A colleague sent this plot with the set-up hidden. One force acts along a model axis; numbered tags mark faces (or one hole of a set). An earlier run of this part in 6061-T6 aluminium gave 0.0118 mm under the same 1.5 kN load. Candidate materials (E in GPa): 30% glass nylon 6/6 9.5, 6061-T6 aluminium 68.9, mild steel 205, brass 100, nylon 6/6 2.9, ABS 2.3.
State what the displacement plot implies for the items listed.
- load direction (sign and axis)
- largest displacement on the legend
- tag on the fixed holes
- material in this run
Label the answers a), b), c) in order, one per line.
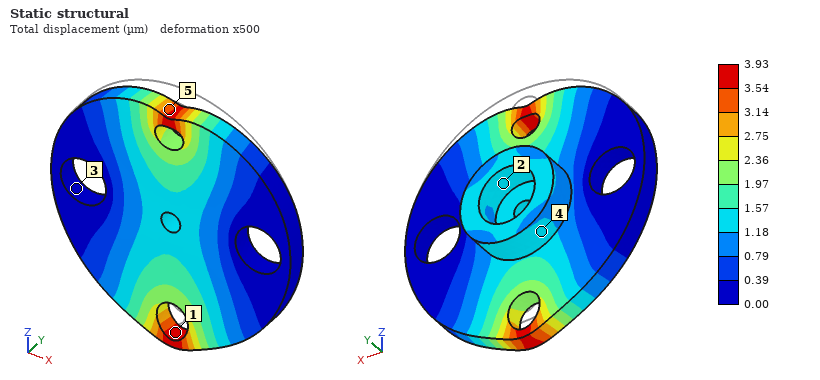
a) -Z
b) 3.93 µm
c) 3
d) mild steel
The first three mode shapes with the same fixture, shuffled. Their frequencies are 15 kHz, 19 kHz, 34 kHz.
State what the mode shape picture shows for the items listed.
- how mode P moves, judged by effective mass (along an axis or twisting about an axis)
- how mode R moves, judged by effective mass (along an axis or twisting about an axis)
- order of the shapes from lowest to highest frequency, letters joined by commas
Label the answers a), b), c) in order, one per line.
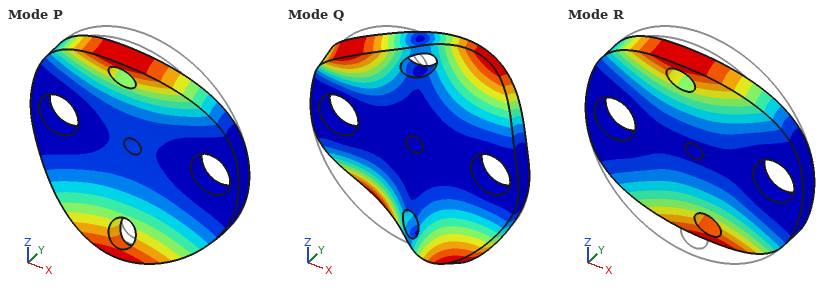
a) along Y
b) twisting about X
c) R, P, Q
